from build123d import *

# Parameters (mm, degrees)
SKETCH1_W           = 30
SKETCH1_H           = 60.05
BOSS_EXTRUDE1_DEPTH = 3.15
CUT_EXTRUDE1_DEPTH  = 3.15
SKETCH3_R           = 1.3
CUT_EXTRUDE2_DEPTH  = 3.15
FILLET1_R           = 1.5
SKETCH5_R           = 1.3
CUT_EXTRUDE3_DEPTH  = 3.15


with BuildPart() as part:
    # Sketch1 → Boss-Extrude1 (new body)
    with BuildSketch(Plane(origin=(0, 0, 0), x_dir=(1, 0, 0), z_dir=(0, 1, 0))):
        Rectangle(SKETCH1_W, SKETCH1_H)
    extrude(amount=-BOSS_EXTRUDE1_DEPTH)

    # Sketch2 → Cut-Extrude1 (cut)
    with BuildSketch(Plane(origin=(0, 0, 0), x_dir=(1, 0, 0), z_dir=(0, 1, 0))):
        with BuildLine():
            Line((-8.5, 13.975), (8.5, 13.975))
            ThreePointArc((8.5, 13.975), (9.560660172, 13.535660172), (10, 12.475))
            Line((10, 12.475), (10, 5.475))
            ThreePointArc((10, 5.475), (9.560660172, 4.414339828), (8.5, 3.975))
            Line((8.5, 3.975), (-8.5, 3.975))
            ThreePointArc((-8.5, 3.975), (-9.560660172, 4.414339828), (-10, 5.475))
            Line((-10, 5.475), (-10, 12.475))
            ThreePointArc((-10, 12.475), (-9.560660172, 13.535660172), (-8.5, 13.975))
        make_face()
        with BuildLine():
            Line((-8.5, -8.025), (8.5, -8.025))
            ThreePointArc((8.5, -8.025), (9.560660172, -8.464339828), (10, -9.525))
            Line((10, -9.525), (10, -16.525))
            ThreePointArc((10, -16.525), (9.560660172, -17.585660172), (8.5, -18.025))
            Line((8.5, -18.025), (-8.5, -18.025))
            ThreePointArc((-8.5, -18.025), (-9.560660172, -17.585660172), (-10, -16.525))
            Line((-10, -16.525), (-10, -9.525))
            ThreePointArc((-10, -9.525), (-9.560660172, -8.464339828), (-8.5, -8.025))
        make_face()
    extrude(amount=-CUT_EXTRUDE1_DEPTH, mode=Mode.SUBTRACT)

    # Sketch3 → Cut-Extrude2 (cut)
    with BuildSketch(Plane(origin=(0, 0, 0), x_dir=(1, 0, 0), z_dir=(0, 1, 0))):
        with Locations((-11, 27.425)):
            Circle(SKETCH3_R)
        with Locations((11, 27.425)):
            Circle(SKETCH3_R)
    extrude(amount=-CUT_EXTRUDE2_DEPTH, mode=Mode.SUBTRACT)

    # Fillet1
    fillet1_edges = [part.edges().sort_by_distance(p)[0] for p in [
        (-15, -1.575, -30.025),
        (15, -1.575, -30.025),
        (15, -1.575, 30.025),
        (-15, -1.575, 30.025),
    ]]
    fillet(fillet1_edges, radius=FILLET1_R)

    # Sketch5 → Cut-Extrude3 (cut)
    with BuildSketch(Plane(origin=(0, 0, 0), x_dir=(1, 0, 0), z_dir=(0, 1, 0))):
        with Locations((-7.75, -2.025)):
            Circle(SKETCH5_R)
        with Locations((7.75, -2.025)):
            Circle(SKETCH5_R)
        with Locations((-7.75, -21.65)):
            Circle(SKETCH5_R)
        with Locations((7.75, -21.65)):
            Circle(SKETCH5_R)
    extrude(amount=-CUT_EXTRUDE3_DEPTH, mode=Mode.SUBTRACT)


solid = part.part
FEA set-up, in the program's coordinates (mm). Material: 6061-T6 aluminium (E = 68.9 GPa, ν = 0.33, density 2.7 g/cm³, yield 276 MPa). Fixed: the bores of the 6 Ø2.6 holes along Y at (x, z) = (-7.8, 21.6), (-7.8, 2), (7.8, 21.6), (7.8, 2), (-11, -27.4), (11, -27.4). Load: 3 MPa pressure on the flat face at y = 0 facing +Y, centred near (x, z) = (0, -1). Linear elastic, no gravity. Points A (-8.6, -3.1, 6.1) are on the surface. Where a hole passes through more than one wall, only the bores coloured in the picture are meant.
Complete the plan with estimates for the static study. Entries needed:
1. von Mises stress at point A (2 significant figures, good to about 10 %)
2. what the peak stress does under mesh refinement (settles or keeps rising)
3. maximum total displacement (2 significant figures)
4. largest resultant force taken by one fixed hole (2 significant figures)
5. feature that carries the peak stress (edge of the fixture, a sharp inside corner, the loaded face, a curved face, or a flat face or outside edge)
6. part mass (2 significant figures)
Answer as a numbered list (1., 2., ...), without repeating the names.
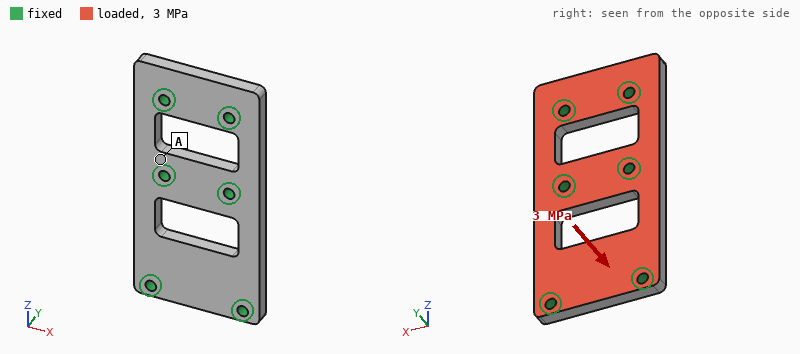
1. 25 MPa
2. keeps rising
3. 70 µm
4. 770 N
5. edge of the fixture
6. 12 g
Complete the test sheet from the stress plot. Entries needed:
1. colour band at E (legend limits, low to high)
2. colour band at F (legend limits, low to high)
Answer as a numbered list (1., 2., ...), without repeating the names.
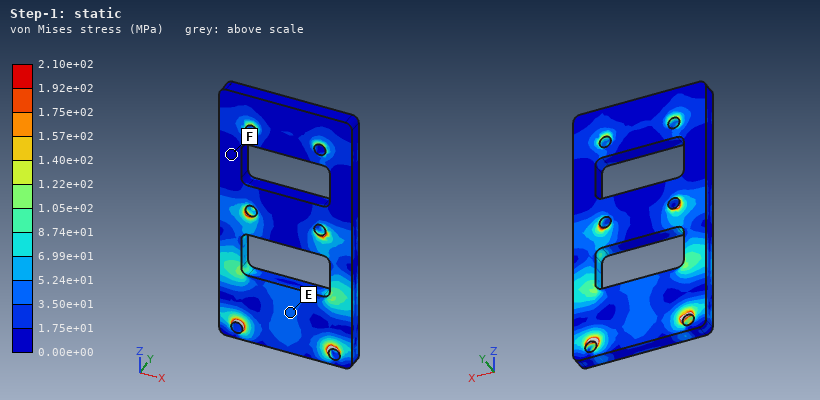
1. 3.50e+01 to 5.24e+01 MPa
2. 0.00e+00 to 1.75e+01 MPa
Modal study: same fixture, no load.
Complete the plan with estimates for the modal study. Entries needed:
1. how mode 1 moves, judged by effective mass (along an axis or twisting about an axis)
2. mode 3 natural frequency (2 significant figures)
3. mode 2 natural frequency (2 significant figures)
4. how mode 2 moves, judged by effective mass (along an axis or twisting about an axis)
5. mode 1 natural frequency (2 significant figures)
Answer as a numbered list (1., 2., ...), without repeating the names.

1. along Y
2. 25 kHz
3. 20 kHz
4. twisting about Z
5. 15 kHz
